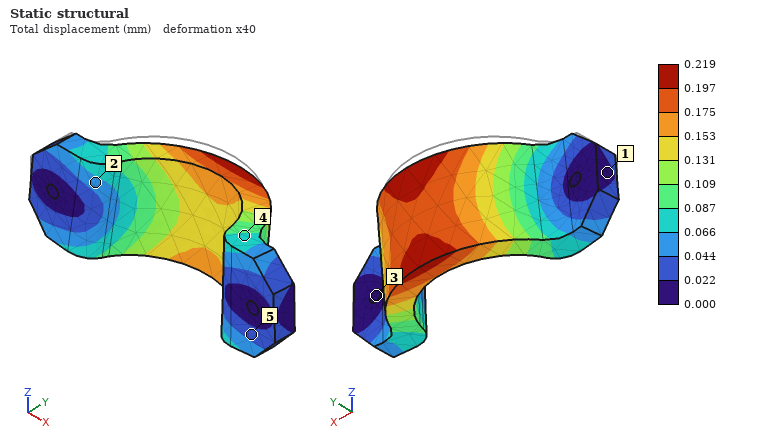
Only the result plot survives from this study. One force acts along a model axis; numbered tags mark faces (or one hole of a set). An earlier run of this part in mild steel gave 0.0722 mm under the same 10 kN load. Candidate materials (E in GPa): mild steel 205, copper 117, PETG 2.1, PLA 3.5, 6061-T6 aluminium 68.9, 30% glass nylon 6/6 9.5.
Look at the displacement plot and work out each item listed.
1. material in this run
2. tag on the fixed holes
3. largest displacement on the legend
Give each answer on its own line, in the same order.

6061-T6 aluminium
3
0.219 mm
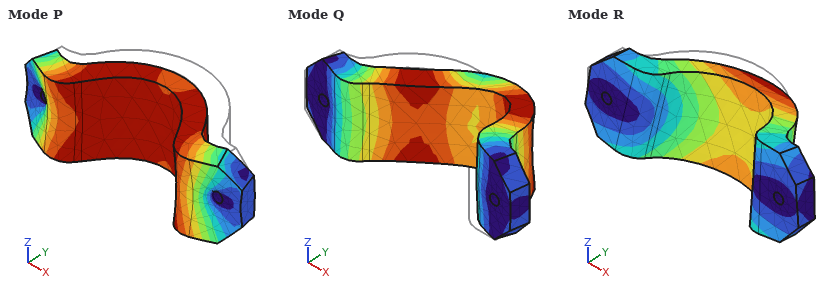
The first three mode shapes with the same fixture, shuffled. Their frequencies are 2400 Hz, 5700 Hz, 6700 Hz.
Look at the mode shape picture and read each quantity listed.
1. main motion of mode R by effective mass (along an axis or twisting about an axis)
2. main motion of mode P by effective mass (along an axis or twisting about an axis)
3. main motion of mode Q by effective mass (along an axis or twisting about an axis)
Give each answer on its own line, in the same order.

along Z
along Y
along X
